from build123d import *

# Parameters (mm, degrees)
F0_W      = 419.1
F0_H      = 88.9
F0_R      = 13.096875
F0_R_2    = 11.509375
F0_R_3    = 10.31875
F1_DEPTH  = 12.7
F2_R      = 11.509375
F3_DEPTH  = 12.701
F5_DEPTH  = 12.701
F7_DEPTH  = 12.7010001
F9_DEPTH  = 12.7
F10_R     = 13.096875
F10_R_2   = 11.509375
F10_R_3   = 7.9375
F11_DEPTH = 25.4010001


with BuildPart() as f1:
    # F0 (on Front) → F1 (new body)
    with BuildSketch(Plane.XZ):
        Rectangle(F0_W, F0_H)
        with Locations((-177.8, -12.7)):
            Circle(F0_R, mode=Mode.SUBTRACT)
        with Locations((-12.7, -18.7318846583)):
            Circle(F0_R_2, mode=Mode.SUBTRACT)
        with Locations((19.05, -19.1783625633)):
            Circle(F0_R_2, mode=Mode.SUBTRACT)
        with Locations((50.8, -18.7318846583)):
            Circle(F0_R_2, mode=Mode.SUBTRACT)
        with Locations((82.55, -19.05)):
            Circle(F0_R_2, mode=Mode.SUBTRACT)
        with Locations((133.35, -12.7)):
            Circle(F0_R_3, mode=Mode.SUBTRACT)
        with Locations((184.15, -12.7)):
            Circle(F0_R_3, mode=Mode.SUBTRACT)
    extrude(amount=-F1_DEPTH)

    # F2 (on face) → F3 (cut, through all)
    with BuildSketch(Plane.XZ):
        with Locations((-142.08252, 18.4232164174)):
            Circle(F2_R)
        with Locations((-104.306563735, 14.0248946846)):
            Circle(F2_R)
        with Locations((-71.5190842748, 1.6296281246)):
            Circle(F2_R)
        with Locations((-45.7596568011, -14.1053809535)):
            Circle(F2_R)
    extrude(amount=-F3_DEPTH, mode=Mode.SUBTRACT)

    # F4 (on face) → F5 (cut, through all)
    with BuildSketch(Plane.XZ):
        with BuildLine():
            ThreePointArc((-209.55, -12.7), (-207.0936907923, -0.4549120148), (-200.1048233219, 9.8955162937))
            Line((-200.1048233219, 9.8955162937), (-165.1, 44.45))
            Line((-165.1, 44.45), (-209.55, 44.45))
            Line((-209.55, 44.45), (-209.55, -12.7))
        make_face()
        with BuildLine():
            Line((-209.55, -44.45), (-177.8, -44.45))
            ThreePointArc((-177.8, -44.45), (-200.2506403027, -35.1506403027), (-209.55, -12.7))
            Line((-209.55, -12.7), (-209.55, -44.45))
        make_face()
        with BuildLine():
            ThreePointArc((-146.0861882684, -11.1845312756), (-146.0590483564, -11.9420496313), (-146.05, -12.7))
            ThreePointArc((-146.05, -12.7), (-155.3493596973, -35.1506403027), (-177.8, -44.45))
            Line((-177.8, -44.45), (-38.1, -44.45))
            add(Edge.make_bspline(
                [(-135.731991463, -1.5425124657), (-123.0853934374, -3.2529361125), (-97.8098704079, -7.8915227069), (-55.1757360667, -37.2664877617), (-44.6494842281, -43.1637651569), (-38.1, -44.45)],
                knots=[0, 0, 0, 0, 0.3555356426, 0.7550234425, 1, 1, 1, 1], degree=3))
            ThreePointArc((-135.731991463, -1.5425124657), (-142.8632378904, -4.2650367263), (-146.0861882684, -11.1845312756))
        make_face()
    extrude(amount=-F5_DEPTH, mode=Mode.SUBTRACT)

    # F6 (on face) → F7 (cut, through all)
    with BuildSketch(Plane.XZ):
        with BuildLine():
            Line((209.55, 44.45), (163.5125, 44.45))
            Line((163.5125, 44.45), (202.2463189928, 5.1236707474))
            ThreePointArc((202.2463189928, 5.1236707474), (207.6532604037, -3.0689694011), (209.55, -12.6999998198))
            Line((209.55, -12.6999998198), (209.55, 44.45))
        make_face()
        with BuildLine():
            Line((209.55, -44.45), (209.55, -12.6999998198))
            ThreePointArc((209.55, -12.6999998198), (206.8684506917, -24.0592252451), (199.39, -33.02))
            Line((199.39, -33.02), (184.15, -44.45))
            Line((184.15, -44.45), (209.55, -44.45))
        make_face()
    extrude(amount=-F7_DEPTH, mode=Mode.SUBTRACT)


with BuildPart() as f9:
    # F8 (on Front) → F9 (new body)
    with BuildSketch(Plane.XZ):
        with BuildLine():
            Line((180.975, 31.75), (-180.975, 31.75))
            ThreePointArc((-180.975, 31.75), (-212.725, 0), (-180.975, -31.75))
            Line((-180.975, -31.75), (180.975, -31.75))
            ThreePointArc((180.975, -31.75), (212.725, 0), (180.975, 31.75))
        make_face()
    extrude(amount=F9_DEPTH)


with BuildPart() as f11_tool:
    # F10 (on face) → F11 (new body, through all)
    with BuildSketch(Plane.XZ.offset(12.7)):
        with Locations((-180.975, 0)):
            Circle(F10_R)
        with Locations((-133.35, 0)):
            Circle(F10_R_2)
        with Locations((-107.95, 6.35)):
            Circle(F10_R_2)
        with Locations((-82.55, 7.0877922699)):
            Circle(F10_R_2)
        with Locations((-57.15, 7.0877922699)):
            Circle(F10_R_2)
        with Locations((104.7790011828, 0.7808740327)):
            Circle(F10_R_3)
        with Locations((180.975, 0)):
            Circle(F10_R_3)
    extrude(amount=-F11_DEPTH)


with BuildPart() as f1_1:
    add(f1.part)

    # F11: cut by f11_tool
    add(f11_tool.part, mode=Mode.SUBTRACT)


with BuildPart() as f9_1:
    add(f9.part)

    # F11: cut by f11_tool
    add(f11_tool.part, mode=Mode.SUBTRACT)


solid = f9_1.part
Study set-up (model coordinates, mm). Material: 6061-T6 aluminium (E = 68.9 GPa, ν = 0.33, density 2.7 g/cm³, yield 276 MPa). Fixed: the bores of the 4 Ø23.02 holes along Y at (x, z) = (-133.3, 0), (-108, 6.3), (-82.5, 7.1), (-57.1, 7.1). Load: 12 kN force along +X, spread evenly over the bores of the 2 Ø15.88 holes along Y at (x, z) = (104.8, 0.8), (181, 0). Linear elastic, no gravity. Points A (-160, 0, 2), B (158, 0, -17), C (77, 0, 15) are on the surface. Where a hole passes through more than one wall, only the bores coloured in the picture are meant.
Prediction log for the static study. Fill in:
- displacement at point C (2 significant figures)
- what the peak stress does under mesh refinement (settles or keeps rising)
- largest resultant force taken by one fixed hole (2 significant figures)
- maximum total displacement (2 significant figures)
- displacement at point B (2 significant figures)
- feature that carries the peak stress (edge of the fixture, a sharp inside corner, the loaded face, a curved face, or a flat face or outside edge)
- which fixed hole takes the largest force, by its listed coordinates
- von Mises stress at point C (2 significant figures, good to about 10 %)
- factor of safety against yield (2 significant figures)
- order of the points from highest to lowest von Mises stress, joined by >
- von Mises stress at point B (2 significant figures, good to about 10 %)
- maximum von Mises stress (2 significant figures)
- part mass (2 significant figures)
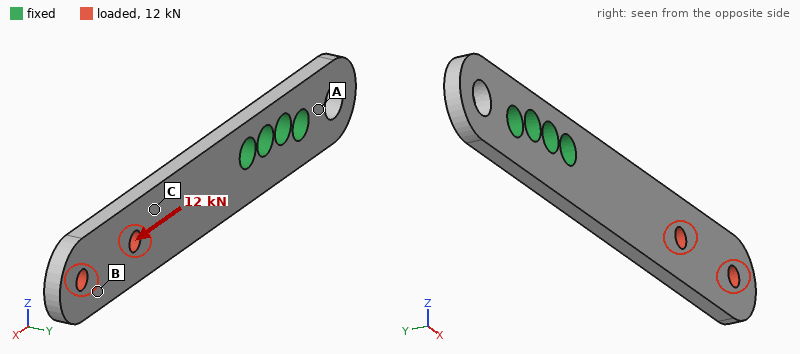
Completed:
30 µm
settles
9.7 kN
52 µm
47 µm
the loaded face
(-57.1, 7.1)
16 MPa
6.9
C > B > A
8.1 MPa
40 MPa
810 g
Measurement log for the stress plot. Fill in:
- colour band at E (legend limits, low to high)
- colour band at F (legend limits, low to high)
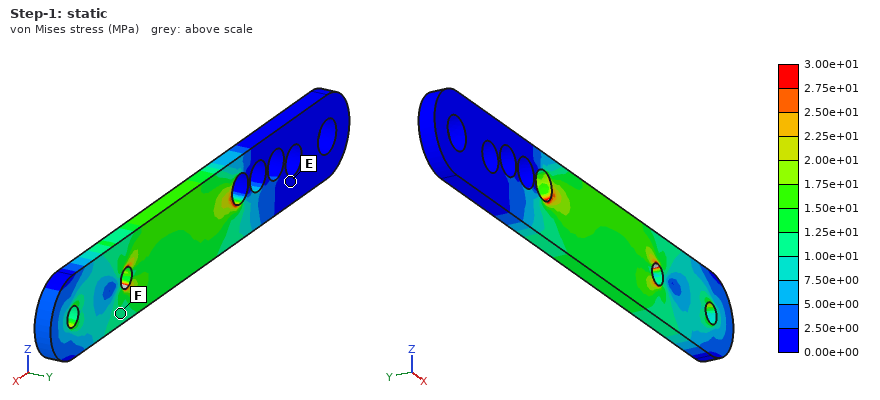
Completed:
0.00e+00 to 2.50e+00 MPa
1.00e+01 to 1.25e+01 MPa
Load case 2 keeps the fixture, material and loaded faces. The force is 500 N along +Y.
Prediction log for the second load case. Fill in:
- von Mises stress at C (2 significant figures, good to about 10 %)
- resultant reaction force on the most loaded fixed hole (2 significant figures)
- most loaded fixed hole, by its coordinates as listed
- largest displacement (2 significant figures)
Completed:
20 MPa
1.0 kN
(-57.1, 7.1)
2.5 mm
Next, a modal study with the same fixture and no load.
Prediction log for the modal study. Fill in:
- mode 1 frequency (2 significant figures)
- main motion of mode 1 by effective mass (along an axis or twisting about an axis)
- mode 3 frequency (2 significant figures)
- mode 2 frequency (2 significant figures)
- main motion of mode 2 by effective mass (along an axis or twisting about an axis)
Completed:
160 Hz
along Y
960 Hz
680 Hz
along Z
